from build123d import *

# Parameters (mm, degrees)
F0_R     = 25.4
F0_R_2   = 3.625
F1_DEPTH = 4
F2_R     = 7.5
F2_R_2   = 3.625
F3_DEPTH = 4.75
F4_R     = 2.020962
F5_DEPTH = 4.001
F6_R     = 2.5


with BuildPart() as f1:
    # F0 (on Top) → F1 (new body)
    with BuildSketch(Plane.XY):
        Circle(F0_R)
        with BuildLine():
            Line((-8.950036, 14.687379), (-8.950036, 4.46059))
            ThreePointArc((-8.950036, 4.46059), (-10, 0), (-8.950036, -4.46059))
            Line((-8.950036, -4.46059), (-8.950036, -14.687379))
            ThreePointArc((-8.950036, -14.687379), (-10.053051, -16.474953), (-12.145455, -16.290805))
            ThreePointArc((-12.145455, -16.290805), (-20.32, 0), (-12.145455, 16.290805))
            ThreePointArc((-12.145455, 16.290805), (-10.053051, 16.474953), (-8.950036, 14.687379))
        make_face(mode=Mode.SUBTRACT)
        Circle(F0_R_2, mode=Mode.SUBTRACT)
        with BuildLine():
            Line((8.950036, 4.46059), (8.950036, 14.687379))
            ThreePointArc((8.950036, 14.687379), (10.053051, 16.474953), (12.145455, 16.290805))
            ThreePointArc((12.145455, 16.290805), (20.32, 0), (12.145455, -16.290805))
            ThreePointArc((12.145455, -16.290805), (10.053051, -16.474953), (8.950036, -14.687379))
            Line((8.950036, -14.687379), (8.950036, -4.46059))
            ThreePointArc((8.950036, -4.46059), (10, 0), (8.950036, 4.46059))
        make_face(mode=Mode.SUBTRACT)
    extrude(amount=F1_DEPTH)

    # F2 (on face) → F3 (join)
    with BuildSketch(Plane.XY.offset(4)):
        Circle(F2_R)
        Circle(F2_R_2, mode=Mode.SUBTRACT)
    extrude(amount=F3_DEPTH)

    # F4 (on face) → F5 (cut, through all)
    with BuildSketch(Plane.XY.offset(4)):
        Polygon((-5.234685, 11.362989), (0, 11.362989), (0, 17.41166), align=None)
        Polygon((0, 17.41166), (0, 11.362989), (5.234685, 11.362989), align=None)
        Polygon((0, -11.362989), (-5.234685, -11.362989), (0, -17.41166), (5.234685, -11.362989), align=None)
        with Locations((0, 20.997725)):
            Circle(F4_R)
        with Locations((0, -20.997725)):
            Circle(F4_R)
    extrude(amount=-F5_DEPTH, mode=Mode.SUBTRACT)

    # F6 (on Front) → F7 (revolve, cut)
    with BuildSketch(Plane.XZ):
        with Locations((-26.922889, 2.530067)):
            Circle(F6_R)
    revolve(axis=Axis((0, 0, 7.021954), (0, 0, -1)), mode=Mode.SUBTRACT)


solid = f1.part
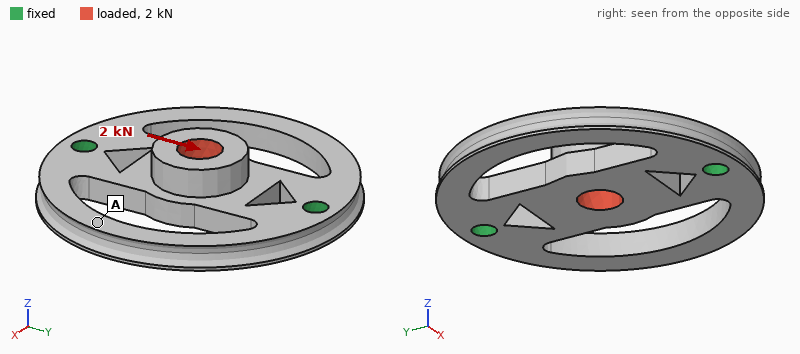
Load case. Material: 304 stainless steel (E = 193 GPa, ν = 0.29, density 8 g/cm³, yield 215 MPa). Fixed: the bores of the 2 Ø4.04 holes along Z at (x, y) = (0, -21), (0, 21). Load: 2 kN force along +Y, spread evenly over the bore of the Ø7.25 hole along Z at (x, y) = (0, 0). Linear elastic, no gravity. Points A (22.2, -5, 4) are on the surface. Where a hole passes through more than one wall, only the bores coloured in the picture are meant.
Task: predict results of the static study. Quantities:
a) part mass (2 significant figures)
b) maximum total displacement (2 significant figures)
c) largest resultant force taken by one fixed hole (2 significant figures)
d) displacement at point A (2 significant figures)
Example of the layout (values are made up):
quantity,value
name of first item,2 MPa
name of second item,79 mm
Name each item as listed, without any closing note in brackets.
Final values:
quantity,value
part mass,44 g
maximum total displacement,6.8 µm
largest resultant force taken by one fixed hole,1.0 kN
displacement at point A,2.7 µm
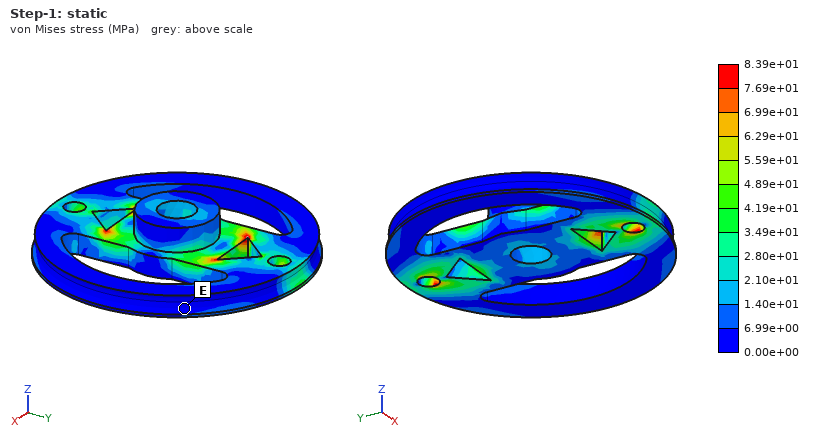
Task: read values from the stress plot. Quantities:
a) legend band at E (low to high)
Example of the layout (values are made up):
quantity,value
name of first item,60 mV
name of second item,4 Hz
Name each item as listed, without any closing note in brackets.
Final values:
quantity,value
legend band at E,0.00e+00 to 6.99e+00 MPa
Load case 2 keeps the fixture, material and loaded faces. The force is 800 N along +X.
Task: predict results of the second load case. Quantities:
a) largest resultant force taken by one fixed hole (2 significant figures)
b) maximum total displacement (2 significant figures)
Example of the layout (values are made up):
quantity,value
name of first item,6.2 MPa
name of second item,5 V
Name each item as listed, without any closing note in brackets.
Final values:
quantity,value
largest resultant force taken by one fixed hole,400 N
maximum total displacement,9.6 µm
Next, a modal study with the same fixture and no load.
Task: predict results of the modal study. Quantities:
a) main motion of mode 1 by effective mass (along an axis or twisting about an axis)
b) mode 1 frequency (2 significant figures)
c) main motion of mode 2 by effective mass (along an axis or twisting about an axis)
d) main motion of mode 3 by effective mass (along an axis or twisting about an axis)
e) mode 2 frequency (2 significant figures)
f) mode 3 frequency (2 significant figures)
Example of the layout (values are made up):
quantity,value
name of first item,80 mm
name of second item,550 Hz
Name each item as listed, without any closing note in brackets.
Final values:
quantity,value
main motion of mode 1 by effective mass,twisting about Y
mode 1 frequency,4400 Hz
main motion of mode 2 by effective mass,along Z
main motion of mode 3 by effective mass,along Z
mode 2 frequency,4700 Hz
mode 3 frequency,9700 Hz
